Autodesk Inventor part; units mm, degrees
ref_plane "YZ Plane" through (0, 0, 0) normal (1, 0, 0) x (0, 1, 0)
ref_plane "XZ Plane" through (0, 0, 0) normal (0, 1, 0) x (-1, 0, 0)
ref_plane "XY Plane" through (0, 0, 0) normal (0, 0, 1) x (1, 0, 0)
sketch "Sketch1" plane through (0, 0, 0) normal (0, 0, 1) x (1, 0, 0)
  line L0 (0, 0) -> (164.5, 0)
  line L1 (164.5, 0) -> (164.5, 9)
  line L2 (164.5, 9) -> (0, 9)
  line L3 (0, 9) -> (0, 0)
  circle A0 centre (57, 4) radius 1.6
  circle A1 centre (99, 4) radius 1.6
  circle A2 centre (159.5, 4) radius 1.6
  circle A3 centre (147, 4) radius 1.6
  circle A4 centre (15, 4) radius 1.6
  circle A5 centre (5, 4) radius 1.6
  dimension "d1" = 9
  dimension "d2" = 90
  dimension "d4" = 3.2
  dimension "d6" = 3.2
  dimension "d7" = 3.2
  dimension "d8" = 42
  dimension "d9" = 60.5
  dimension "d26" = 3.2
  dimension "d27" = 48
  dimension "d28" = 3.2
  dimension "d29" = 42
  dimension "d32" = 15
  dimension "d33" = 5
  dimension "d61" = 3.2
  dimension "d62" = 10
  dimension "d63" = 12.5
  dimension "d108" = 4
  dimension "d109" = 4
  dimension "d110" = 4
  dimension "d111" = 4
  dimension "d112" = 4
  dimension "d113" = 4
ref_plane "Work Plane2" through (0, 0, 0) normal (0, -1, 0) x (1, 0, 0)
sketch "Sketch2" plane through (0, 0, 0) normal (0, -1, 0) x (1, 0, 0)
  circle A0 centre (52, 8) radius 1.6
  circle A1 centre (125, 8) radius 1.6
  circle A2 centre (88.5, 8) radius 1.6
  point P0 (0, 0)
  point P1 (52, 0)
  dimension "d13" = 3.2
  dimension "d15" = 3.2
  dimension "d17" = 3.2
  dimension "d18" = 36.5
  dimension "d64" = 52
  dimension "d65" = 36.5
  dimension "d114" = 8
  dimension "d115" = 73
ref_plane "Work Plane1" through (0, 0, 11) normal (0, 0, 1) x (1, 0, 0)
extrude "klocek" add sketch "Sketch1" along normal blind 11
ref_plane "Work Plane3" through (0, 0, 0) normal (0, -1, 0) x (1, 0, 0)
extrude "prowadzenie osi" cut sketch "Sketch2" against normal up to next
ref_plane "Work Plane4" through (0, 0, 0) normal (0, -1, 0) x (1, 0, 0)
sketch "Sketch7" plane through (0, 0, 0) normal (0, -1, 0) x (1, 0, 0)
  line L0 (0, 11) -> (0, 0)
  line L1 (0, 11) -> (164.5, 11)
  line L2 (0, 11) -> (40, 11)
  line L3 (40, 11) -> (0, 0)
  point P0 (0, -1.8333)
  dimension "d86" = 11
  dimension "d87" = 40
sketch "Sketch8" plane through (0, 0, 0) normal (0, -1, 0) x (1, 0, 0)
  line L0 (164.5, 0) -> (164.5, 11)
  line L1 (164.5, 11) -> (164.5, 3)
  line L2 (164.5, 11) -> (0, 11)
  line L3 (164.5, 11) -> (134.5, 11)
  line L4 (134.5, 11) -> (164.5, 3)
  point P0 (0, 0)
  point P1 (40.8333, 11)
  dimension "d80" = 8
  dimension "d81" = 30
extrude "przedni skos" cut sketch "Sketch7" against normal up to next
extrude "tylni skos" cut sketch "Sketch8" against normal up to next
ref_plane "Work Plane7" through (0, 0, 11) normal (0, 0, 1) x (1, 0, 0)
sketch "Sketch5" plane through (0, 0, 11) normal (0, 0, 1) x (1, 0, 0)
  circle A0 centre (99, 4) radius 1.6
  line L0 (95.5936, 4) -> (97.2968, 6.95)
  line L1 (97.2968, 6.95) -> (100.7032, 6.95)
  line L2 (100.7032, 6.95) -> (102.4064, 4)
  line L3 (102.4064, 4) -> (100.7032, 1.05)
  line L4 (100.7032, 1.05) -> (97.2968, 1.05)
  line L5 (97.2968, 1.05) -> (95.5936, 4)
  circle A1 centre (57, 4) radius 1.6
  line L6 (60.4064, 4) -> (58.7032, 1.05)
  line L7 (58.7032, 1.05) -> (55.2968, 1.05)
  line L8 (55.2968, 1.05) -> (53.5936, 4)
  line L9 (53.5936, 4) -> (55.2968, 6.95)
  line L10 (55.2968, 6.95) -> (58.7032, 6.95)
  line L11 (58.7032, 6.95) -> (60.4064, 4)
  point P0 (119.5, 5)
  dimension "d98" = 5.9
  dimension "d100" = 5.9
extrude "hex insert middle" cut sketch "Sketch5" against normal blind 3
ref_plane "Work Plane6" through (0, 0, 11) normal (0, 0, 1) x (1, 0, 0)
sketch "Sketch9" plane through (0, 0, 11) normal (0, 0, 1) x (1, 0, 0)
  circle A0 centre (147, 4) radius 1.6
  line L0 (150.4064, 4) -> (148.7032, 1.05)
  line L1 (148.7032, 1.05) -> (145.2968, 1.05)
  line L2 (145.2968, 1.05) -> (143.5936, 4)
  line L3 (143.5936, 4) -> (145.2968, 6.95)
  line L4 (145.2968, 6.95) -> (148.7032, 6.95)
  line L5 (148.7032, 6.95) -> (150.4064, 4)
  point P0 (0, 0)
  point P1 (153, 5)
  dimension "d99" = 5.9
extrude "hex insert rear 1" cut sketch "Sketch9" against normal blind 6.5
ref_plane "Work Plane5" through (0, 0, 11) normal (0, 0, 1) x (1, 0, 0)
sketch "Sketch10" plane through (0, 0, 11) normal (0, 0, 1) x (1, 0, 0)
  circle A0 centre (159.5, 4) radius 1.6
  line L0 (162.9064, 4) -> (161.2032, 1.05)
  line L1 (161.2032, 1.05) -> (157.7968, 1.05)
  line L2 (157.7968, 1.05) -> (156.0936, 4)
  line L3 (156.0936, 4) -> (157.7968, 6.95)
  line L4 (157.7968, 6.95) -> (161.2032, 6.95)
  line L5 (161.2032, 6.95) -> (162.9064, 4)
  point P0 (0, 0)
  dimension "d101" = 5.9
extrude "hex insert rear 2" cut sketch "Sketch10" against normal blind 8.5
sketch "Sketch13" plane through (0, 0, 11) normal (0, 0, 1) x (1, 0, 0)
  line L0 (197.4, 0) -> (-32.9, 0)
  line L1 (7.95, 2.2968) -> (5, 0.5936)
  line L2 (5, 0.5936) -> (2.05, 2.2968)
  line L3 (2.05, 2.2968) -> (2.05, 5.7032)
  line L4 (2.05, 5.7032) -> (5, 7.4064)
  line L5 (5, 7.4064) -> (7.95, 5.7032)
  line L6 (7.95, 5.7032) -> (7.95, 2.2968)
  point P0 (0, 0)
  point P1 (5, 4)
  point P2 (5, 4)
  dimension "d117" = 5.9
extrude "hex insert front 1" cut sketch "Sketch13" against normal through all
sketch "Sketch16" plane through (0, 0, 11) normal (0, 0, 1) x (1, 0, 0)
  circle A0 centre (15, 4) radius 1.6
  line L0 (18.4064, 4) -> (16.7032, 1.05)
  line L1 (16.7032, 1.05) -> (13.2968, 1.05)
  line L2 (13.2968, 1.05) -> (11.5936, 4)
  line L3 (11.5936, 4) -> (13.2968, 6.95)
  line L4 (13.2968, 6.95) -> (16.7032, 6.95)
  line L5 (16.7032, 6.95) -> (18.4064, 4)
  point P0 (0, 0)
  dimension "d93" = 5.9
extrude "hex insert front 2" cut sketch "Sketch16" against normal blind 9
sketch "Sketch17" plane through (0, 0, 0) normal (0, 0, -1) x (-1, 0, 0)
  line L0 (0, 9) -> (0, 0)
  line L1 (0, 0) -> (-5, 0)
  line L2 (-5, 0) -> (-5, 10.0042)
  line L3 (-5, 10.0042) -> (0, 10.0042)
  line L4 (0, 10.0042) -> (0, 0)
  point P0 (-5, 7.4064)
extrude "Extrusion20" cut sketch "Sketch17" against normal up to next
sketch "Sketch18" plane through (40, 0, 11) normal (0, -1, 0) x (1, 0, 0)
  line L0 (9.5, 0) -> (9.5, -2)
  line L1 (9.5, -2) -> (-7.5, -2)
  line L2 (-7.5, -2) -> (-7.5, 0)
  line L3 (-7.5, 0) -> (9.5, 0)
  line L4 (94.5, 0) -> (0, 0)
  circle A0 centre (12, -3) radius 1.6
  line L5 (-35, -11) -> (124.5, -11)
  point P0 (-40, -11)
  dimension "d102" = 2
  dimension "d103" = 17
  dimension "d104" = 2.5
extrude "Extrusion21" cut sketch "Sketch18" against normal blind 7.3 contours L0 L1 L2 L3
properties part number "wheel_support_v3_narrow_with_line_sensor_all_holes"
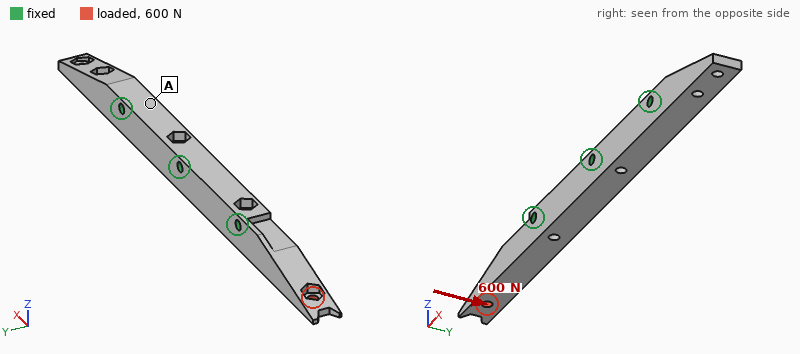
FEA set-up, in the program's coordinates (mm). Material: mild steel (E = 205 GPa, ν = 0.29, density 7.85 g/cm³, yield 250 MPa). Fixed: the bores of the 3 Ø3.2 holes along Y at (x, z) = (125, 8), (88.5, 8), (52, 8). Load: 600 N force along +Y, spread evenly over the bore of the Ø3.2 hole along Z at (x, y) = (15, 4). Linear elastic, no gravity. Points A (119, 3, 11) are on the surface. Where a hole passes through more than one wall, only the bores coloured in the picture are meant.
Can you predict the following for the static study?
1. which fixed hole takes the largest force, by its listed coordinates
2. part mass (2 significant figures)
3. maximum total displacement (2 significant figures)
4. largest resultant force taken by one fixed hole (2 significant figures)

(52, 8)
95 g
0.14 mm
710 N
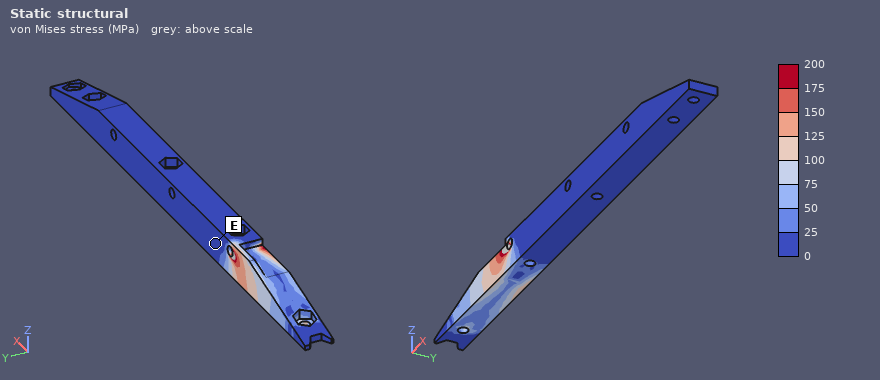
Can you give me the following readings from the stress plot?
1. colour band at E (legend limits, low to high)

0 to 25 MPa
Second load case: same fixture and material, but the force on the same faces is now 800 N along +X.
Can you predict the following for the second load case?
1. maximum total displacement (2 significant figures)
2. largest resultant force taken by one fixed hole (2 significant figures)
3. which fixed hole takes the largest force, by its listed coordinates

40 µm
550 N
(52, 8)
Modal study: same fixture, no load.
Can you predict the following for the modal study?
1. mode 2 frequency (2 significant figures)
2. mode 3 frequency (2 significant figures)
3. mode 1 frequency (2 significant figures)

5400 Hz
6600 Hz
4900 Hz
